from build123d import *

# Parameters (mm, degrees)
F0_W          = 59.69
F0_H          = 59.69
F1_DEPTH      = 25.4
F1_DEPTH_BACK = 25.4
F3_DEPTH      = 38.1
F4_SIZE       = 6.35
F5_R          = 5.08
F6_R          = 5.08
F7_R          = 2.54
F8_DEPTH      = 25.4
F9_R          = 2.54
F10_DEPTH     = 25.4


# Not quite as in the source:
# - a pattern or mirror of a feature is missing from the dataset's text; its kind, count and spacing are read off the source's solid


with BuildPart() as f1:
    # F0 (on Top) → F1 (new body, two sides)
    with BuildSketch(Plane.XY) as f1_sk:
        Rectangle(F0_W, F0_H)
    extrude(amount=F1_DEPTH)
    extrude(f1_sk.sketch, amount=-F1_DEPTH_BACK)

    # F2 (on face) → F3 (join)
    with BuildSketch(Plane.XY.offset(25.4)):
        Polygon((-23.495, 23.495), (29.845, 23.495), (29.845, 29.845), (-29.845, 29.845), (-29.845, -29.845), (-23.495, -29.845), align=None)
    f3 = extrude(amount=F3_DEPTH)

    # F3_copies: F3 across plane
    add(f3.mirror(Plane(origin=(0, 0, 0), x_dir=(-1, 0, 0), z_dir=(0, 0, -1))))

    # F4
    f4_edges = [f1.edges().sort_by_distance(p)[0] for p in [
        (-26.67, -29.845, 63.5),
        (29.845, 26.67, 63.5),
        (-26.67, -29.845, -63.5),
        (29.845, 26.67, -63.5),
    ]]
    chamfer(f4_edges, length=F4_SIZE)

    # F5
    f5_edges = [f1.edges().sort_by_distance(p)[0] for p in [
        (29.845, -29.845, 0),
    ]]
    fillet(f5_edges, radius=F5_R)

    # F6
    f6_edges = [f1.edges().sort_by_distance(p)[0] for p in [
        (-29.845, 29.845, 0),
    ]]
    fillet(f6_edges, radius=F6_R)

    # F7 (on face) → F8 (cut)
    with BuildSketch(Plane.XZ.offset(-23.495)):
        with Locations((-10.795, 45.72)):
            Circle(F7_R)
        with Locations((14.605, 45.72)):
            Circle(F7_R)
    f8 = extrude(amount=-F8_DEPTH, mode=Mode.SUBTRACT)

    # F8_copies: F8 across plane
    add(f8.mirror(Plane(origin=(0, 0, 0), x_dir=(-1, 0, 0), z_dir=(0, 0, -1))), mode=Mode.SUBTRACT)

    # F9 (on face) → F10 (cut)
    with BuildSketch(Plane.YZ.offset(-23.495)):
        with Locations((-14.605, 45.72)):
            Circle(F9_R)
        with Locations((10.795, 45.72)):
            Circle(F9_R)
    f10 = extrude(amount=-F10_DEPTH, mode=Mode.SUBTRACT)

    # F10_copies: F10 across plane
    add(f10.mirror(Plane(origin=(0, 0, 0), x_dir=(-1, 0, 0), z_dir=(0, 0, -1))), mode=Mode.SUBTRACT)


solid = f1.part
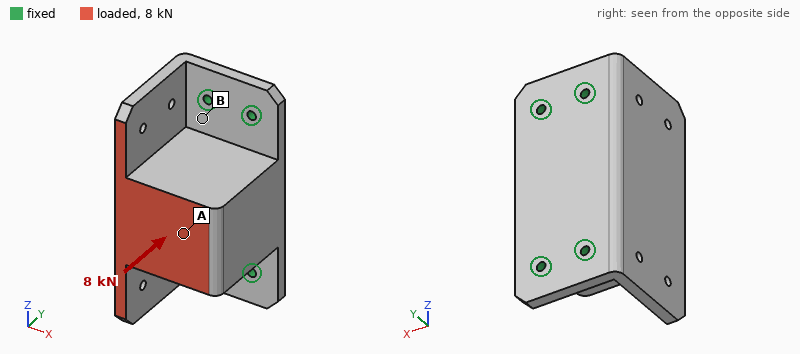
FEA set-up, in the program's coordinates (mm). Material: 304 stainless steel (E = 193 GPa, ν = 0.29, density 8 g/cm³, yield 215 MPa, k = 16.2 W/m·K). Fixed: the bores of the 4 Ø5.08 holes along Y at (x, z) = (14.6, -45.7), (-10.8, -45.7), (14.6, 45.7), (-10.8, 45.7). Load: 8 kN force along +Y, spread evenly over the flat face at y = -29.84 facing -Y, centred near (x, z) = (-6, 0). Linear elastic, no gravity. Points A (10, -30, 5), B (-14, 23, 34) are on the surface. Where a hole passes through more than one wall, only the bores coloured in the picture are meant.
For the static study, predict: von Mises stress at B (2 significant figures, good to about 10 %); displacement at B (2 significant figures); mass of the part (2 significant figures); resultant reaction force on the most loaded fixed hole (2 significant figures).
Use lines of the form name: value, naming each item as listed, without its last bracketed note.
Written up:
von Mises stress at B: 31 MPa
displacement at B: 8.6 µm
mass of the part: 1.9 kg
resultant reaction force on the most loaded fixed hole: 3.0 kN
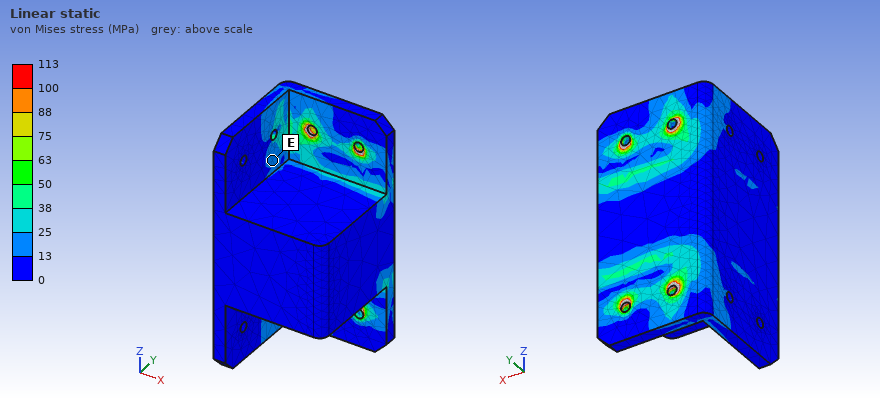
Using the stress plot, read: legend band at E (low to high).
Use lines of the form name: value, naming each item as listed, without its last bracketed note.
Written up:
legend band at E: 13 to 25 MPa
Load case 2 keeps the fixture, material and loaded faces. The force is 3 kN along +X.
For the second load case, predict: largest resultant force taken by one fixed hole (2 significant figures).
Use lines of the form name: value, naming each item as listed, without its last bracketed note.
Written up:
largest resultant force taken by one fixed hole: 2.9 kN
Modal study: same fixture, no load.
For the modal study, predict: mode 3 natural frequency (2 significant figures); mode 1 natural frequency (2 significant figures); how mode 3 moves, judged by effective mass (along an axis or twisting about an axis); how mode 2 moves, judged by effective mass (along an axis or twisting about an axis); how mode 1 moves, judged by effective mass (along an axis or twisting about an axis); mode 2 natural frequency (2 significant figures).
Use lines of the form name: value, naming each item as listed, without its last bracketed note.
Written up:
mode 3 natural frequency: 2900 Hz
mode 1 natural frequency: 1300 Hz
how mode 3 moves, judged by effective mass: along Z
how mode 2 moves, judged by effective mass: along Y
how mode 1 moves, judged by effective mass: along X
mode 2 natural frequency: 2800 Hz
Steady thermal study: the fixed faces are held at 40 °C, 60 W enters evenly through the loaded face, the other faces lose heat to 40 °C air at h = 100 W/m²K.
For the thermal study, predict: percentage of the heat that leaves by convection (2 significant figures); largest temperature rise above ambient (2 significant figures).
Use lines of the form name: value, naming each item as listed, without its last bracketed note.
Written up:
percentage of the heat that leaves by convection: 90 %
largest temperature rise above ambient: 53 K
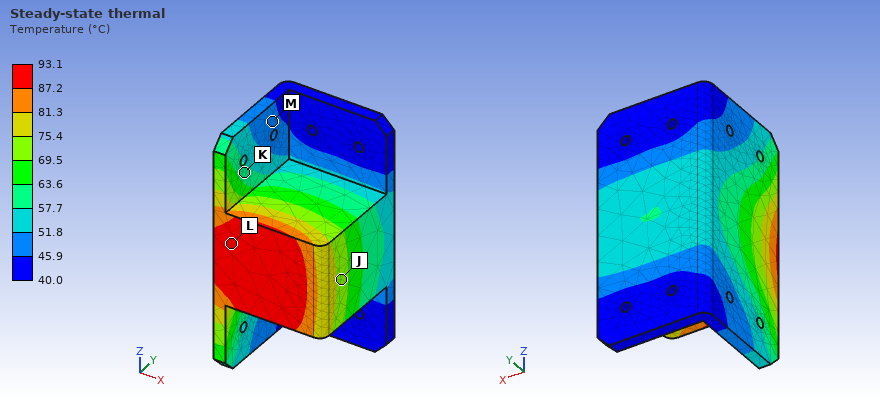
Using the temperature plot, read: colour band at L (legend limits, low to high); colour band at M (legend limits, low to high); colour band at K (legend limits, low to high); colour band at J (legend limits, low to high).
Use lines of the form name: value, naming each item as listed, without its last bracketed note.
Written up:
colour band at L: 87.2 to 93.1 °C
colour band at M: 45.9 to 51.8 °C
colour band at K: 57.7 to 63.6 °C
colour band at J: 69.5 to 75.4 °C
